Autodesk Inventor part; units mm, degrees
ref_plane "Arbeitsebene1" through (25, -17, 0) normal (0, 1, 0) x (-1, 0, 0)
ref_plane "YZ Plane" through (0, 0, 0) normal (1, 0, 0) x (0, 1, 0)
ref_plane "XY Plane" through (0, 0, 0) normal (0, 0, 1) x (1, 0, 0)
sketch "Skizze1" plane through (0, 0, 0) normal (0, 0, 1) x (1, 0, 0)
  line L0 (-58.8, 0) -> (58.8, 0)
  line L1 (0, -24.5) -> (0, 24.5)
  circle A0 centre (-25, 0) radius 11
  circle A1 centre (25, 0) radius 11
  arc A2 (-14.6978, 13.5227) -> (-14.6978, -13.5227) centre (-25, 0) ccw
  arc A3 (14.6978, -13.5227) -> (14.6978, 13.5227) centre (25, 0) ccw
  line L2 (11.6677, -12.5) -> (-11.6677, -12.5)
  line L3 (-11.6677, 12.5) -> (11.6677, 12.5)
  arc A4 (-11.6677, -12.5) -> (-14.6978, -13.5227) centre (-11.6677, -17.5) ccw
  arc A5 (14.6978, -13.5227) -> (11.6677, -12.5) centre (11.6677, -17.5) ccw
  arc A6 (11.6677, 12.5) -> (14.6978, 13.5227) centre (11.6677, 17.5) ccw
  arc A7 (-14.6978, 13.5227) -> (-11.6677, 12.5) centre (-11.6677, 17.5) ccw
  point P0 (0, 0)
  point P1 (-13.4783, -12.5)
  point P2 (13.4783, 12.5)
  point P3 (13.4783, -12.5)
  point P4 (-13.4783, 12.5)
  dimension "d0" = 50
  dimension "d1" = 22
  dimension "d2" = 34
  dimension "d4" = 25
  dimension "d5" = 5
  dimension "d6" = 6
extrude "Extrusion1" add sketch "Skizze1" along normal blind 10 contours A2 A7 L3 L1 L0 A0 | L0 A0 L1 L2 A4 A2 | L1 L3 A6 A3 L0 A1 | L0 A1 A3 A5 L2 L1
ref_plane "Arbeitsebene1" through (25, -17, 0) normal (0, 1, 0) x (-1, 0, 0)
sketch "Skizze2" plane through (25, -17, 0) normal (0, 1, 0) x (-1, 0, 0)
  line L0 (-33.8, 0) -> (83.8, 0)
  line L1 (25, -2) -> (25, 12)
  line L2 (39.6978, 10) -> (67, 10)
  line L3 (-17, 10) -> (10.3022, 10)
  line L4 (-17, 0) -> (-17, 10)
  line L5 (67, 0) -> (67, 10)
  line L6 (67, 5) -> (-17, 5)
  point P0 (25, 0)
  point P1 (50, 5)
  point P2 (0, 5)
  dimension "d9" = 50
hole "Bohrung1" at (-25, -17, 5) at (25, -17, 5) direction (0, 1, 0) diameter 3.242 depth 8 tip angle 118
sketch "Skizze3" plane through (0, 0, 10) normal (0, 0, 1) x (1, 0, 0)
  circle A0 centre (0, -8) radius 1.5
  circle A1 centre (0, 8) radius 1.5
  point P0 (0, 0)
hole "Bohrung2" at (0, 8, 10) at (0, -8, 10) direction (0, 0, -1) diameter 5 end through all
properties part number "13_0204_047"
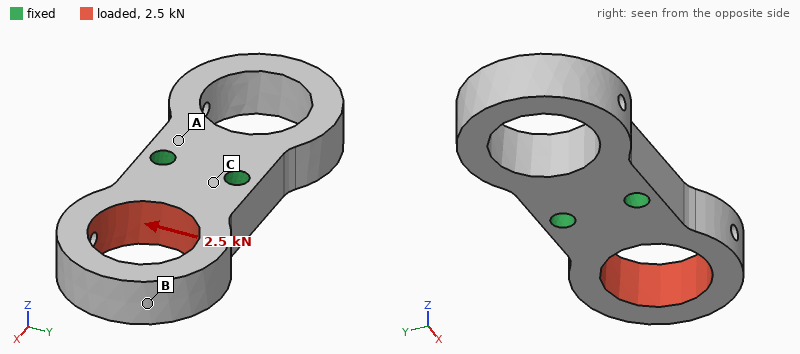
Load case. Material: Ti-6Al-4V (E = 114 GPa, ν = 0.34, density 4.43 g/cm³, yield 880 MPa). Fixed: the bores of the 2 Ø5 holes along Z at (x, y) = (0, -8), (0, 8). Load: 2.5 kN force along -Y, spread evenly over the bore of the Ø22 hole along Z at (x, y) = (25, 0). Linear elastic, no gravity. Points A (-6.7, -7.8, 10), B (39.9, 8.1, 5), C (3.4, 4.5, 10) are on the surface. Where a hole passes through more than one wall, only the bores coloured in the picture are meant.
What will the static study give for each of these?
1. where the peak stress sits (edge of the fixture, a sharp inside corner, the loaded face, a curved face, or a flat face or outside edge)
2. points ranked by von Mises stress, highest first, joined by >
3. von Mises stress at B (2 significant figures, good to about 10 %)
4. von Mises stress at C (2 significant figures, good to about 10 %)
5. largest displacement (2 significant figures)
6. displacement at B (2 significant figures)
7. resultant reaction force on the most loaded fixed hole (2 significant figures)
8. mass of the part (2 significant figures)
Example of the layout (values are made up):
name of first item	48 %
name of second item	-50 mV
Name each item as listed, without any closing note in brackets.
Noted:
where the peak stress sits	a curved face
points ranked by von Mises stress, highest first, joined by >	B > C > A
von Mises stress at B	38 MPa
von Mises stress at C	24 MPa
largest displacement	76 µm
displacement at B	76 µm
resultant reaction force on the most loaded fixed hole	3.5 kN
mass of the part	66 g
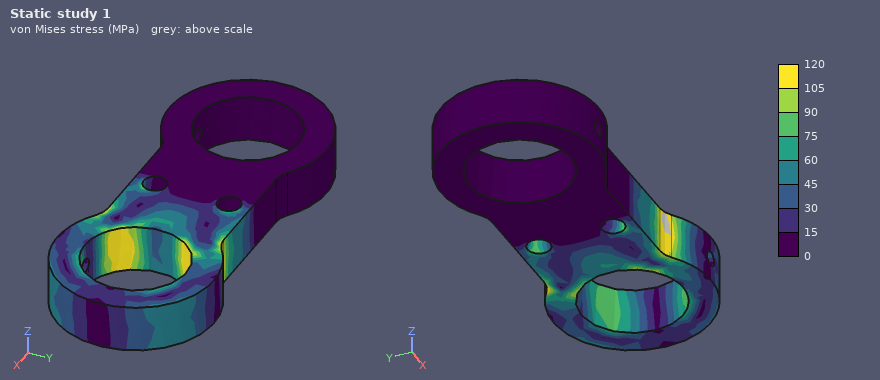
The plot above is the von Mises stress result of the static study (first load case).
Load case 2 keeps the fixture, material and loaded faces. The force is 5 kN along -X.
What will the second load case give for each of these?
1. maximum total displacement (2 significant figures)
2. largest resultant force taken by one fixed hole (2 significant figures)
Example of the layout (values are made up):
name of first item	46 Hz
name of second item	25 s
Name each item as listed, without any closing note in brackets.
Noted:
maximum total displacement	24 µm
largest resultant force taken by one fixed hole	2.5 kN
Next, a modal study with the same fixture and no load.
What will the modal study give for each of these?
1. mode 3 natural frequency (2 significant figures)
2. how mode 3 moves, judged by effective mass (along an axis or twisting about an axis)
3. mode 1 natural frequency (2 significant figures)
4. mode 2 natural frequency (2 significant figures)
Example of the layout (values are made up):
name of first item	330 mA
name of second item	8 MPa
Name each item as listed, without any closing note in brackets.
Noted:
mode 3 natural frequency	6500 Hz
how mode 3 moves, judged by effective mass	twisting about Z
mode 1 natural frequency	4600 Hz
mode 2 natural frequency	4800 Hz
